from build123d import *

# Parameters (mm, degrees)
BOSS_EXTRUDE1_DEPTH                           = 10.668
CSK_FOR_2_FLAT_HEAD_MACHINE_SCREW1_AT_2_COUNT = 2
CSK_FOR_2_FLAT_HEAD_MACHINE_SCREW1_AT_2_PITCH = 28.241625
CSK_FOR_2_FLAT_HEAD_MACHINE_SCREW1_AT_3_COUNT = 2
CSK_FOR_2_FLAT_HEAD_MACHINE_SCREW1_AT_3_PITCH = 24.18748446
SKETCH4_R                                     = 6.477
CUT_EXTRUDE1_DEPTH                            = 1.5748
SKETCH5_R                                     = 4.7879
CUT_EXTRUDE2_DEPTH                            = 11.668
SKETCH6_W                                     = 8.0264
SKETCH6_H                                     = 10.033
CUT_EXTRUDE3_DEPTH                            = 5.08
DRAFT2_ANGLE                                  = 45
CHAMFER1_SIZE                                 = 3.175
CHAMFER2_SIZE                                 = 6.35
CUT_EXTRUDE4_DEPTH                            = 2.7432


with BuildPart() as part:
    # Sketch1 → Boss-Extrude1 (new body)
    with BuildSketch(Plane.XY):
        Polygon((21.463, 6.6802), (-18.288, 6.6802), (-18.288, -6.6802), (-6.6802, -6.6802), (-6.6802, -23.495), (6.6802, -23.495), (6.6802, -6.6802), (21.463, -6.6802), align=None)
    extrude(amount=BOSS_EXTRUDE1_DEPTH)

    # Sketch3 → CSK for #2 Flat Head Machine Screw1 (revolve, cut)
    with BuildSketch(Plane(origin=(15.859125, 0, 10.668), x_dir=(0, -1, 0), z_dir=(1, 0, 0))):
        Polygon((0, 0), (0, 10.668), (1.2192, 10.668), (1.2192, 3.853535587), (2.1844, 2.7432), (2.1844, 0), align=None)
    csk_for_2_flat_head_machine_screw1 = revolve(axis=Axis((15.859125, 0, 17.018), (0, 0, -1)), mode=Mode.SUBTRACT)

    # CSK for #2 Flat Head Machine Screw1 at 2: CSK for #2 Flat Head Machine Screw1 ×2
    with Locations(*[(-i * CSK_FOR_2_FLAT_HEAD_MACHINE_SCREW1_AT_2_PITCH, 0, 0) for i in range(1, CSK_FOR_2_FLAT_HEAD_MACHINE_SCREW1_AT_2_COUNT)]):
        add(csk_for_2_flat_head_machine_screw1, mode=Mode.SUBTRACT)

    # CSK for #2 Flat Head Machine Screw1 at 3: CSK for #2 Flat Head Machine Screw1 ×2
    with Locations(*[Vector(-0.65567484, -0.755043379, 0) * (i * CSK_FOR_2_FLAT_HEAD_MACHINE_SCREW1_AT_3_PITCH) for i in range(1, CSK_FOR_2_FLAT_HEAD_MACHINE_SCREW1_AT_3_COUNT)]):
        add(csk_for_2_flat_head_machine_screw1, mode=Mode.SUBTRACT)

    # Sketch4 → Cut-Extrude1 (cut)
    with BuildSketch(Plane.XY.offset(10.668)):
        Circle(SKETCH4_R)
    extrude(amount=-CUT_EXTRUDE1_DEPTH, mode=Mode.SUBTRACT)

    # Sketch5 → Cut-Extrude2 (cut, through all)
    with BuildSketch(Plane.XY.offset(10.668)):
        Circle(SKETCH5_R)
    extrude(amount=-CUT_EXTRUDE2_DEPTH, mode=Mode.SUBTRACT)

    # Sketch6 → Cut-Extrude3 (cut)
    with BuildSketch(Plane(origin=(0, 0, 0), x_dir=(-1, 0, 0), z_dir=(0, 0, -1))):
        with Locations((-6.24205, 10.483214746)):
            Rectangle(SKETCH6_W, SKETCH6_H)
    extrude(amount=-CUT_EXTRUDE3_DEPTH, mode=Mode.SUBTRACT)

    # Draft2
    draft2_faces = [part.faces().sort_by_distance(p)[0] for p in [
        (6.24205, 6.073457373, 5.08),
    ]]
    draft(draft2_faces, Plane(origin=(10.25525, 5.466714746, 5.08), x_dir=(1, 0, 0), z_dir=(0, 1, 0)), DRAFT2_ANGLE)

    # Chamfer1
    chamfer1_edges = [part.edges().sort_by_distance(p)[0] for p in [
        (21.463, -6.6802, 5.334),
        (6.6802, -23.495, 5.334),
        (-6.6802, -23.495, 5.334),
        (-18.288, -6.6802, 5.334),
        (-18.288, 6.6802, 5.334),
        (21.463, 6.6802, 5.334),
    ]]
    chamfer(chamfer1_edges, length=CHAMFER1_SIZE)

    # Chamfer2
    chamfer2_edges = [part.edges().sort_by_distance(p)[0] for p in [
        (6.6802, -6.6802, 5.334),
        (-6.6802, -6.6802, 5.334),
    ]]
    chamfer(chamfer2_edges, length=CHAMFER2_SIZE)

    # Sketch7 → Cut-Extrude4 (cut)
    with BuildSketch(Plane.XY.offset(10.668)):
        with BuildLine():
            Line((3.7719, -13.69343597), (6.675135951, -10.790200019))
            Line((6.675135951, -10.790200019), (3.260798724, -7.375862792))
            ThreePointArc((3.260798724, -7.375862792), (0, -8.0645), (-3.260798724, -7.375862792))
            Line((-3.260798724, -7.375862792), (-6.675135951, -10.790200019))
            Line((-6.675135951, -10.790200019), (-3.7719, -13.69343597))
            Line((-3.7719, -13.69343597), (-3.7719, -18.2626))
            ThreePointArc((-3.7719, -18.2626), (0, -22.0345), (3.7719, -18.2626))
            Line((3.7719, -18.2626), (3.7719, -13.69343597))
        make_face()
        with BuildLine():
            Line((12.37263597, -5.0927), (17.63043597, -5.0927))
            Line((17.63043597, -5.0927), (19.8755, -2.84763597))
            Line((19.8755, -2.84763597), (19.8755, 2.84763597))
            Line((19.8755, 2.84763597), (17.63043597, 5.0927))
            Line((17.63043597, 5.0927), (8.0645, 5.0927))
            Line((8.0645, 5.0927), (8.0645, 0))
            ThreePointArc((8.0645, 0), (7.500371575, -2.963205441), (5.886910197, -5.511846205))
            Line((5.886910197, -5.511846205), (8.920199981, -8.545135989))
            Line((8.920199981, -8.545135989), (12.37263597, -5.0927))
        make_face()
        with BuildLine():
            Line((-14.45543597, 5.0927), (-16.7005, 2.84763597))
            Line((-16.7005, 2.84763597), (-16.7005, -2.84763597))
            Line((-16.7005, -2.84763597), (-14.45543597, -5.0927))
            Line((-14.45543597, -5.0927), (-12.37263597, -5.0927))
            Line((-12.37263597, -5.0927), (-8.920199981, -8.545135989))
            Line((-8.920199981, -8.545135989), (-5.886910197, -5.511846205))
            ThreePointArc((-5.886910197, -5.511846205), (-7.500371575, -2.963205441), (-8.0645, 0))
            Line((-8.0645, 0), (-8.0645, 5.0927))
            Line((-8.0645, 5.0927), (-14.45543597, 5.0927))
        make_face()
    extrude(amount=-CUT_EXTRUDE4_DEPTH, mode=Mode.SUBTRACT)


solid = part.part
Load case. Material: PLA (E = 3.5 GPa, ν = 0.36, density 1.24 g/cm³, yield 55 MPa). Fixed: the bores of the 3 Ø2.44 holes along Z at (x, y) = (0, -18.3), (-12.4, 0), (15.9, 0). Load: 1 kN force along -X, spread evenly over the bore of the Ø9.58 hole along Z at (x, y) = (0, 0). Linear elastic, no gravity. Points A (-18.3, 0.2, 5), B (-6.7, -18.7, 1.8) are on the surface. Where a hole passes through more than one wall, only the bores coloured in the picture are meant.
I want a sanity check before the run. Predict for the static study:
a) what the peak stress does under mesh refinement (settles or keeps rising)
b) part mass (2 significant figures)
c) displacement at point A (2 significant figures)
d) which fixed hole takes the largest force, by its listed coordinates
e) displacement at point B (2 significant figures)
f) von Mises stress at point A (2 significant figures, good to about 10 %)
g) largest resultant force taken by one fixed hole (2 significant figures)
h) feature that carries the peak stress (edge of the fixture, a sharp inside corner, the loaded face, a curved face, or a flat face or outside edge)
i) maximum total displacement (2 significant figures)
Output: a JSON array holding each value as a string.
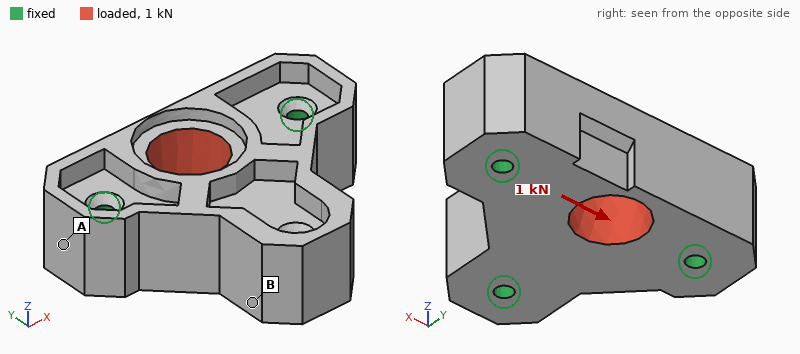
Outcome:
["keeps rising", "7.7 g", "4.6 µm", "(-12.4, 0)", "6.7 µm", "3.9 MPa", "500 N", "edge of the fixture", "27 µm"]
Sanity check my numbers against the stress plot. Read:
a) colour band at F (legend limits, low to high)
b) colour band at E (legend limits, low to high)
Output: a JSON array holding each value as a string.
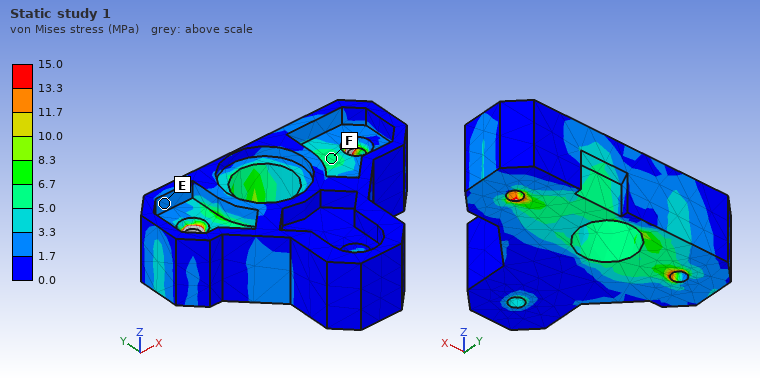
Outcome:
["5.0 to 6.7 MPa", "1.7 to 3.3 MPa"]
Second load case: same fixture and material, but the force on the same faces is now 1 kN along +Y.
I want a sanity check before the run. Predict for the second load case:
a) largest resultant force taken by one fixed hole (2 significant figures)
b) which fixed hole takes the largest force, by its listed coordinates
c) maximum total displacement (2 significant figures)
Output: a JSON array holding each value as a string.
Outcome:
["490 N", "(0, -18.3)", "78 µm"]
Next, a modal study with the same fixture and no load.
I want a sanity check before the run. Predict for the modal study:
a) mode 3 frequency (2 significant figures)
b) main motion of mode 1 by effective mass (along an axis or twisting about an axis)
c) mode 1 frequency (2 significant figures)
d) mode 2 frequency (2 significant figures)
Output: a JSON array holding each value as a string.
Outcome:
["14 kHz", "along Z", "11 kHz", "14 kHz"]
